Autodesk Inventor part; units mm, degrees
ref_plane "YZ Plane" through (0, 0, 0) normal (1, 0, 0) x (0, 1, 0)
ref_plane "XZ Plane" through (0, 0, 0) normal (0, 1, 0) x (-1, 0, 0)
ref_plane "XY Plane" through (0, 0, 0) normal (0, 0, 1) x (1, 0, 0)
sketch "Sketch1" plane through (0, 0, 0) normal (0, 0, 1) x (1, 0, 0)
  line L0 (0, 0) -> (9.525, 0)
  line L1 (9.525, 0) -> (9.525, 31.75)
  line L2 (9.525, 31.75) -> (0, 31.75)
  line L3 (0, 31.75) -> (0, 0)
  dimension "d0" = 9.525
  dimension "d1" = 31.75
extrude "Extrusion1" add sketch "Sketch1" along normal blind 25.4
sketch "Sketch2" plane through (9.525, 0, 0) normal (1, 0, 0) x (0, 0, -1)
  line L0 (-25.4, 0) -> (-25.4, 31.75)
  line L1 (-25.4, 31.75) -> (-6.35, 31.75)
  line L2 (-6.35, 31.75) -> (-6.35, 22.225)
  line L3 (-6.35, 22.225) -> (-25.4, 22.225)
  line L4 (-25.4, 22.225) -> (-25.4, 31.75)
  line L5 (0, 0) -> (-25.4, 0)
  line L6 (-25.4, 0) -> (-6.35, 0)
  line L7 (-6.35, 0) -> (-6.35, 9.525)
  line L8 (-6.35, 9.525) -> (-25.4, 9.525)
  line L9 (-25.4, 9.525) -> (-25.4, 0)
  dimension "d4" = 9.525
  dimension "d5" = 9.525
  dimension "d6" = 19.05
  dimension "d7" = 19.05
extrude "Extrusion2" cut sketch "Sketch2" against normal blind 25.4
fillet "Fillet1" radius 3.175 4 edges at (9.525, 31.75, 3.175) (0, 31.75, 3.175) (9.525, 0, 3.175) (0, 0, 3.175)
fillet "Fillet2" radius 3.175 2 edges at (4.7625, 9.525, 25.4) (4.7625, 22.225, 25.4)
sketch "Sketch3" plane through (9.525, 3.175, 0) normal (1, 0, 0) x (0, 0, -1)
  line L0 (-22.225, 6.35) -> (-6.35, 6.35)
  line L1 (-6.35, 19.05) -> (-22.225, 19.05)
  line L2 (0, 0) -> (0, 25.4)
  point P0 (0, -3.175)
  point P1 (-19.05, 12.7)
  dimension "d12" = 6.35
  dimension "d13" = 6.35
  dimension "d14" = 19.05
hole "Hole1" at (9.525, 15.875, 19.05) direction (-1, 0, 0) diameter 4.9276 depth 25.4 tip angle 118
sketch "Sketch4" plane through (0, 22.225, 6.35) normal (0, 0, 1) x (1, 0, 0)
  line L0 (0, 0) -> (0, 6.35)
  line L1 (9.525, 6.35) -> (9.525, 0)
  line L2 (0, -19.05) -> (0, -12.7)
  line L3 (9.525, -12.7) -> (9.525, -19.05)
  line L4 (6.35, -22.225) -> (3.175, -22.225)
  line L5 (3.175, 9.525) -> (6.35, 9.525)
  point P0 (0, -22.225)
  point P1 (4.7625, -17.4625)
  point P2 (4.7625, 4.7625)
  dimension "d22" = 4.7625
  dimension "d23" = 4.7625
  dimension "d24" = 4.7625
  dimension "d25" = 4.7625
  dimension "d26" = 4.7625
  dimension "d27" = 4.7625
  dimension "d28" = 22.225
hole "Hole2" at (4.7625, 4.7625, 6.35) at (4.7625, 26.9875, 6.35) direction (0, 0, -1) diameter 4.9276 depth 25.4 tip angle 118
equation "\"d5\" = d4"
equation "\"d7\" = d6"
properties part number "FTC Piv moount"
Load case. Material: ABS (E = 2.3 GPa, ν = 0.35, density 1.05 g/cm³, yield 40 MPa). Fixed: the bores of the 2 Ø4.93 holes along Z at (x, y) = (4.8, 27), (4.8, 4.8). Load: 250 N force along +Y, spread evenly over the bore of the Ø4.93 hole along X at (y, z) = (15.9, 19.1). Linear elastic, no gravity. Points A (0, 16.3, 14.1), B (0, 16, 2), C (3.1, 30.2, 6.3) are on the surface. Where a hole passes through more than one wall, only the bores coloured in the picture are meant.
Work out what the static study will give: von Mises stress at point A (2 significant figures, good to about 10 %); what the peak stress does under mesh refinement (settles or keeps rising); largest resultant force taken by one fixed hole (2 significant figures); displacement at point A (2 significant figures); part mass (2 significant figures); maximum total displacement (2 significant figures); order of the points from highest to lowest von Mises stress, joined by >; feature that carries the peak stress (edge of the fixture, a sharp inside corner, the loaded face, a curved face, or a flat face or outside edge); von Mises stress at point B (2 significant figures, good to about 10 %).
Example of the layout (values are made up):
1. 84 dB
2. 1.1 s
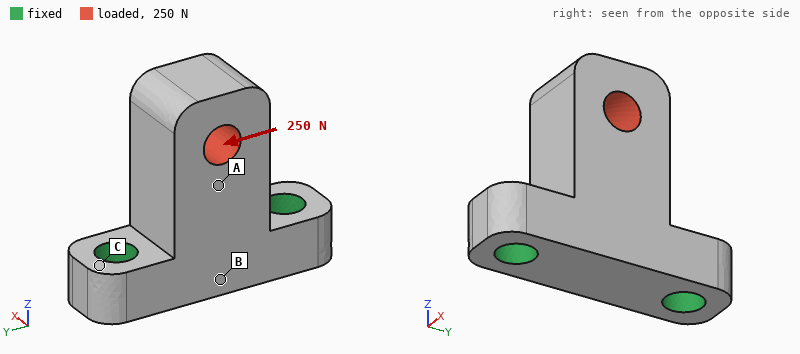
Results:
1. 7.9 MPa
2. keeps rising
3. 270 N
4. 0.085 mm
5. 3.9 g
6. 0.23 mm
7. A > B > C
8. a sharp inside corner
9. 4.7 MPa
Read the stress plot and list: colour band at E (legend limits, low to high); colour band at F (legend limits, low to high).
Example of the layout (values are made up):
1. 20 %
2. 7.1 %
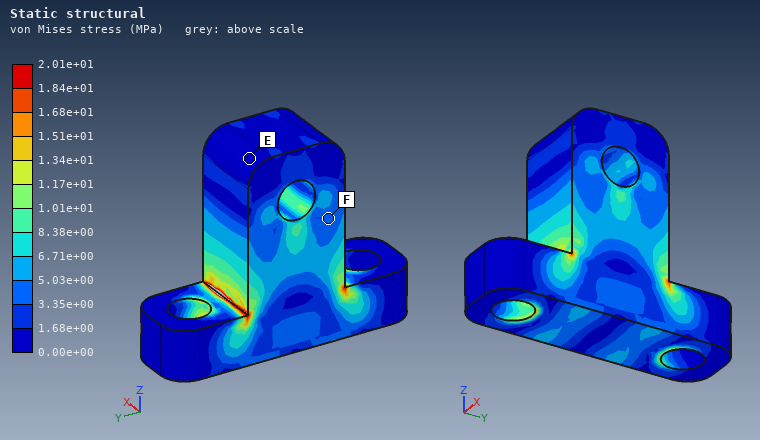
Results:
1. 0.00e+00 to 1.68e+00 MPa
2. 3.35e+00 to 5.03e+00 MPa
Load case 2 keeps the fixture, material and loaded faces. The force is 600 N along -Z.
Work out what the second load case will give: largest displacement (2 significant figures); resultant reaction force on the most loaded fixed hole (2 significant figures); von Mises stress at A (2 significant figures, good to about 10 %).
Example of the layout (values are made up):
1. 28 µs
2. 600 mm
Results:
1. 89 µm
2. 310 N
3. 4.6 MPa
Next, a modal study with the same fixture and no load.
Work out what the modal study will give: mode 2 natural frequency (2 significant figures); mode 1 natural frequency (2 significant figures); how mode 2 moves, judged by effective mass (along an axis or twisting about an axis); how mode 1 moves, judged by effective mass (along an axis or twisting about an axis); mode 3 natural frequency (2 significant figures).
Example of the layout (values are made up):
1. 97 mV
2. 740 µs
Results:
1. 5000 Hz
2. 2800 Hz
3. along Y
4. along X
5. 9300 Hz
